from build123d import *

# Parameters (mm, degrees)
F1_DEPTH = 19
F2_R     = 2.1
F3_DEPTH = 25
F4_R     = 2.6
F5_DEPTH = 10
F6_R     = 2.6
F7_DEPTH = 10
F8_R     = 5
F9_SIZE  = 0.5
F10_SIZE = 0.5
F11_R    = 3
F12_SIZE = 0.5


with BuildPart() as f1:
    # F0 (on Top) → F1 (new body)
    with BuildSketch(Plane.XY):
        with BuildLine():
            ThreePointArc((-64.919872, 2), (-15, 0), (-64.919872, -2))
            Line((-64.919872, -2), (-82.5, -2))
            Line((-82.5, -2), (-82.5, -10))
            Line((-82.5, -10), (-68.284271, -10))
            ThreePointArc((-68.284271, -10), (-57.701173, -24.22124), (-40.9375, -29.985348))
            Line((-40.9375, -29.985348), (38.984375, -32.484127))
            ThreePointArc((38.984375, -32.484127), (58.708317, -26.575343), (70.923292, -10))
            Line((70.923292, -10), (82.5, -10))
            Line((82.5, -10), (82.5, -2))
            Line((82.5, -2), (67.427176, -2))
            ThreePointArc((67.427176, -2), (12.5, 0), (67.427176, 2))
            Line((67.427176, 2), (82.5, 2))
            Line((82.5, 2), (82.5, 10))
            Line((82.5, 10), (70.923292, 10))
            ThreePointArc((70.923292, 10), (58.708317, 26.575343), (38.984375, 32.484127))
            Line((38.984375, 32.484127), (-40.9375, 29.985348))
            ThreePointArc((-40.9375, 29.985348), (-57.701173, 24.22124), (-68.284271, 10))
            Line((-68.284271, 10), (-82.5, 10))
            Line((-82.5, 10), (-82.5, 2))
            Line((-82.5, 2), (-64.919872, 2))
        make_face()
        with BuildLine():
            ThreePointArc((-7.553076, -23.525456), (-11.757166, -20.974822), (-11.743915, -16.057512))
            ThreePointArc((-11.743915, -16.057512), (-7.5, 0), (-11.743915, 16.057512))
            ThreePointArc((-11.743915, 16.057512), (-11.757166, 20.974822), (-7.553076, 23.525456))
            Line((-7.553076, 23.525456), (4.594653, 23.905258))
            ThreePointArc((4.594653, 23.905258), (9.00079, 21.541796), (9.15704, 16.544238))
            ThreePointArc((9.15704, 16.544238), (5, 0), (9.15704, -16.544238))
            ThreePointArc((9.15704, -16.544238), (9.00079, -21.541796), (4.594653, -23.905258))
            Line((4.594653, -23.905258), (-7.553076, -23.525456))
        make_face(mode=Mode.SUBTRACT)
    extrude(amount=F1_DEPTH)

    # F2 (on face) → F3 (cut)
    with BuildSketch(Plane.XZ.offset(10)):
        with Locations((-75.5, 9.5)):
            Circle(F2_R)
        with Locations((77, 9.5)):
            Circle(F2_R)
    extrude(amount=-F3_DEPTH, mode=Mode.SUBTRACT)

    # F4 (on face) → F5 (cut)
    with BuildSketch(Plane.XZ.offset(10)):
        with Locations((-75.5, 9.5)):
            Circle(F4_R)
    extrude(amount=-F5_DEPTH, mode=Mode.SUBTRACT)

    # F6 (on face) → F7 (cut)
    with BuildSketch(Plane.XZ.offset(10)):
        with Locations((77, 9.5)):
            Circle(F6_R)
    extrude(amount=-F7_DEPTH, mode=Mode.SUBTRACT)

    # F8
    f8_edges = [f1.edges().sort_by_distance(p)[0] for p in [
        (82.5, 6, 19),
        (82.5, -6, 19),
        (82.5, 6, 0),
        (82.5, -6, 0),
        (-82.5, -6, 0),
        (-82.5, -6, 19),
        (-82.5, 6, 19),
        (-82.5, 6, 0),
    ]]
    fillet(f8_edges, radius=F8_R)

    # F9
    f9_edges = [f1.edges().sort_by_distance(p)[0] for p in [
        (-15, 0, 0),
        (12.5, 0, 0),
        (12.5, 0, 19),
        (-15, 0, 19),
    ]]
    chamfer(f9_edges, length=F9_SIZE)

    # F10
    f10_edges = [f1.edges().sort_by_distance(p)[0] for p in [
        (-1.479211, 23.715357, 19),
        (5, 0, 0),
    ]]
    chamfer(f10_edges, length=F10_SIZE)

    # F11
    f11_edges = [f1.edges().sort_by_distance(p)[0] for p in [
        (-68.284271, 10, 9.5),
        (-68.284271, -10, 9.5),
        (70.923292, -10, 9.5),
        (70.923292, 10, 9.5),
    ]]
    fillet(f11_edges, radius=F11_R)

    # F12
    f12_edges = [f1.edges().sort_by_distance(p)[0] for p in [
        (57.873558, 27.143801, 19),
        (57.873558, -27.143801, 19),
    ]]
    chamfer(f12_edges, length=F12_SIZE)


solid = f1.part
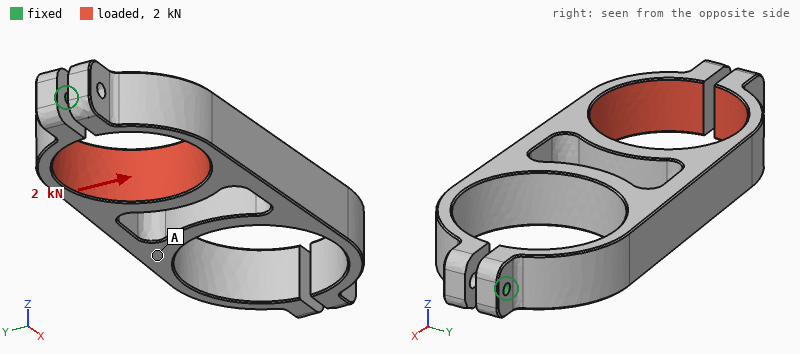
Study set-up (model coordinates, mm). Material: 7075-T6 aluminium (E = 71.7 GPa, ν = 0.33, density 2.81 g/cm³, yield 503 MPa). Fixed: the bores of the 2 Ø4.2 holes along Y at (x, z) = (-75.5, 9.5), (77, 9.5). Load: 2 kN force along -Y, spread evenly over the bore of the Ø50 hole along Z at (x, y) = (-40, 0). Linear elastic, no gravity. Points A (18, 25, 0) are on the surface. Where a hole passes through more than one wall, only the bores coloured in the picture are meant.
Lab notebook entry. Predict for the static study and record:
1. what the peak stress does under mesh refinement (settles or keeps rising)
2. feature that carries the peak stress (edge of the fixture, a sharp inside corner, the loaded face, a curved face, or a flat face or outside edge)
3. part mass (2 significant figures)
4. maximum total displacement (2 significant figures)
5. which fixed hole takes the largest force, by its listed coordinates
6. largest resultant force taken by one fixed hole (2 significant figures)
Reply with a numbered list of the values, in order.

1. keeps rising
2. edge of the fixture
3. 170 g
4. 1.6 mm
5. (-75.5, 9.5)
6. 2.1 kN
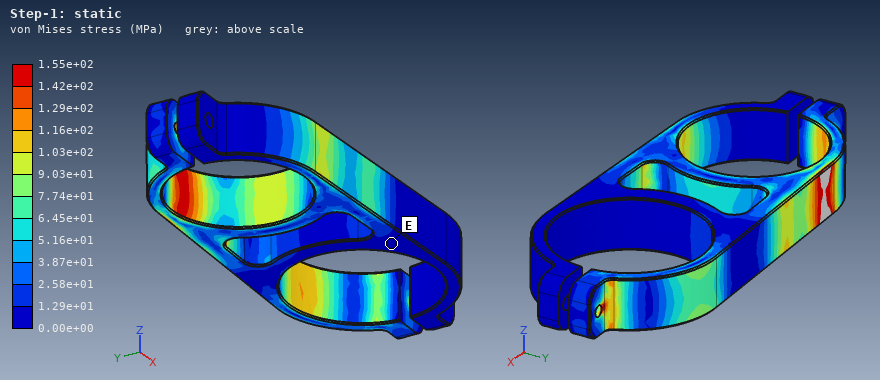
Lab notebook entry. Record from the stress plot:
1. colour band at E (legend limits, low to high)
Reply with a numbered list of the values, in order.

1. 0.00e+00 to 1.29e+01 MPa
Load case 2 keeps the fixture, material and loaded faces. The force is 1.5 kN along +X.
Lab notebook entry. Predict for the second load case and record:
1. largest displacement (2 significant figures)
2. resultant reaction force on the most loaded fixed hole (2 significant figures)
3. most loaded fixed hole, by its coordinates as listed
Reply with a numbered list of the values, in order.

1. 0.71 mm
2. 1.1 kN
3. (-75.5, 9.5)
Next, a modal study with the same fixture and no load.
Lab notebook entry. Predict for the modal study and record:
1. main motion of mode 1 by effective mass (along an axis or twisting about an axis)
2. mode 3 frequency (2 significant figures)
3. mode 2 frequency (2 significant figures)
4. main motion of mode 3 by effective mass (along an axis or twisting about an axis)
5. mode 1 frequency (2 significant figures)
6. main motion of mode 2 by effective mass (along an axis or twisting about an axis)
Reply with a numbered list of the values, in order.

1. along Z
2. 750 Hz
3. 590 Hz
4. twisting about Y
5. 390 Hz
6. along X
